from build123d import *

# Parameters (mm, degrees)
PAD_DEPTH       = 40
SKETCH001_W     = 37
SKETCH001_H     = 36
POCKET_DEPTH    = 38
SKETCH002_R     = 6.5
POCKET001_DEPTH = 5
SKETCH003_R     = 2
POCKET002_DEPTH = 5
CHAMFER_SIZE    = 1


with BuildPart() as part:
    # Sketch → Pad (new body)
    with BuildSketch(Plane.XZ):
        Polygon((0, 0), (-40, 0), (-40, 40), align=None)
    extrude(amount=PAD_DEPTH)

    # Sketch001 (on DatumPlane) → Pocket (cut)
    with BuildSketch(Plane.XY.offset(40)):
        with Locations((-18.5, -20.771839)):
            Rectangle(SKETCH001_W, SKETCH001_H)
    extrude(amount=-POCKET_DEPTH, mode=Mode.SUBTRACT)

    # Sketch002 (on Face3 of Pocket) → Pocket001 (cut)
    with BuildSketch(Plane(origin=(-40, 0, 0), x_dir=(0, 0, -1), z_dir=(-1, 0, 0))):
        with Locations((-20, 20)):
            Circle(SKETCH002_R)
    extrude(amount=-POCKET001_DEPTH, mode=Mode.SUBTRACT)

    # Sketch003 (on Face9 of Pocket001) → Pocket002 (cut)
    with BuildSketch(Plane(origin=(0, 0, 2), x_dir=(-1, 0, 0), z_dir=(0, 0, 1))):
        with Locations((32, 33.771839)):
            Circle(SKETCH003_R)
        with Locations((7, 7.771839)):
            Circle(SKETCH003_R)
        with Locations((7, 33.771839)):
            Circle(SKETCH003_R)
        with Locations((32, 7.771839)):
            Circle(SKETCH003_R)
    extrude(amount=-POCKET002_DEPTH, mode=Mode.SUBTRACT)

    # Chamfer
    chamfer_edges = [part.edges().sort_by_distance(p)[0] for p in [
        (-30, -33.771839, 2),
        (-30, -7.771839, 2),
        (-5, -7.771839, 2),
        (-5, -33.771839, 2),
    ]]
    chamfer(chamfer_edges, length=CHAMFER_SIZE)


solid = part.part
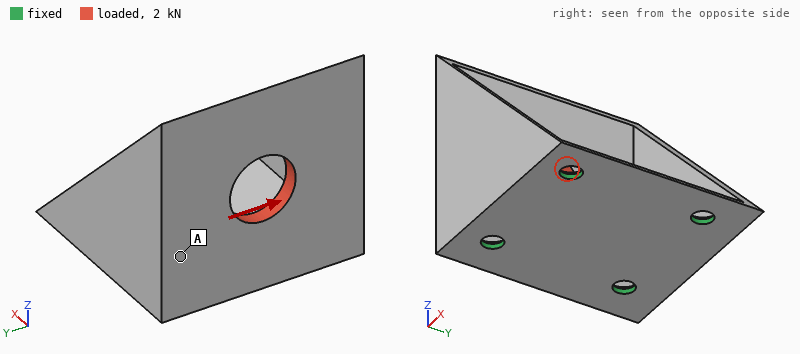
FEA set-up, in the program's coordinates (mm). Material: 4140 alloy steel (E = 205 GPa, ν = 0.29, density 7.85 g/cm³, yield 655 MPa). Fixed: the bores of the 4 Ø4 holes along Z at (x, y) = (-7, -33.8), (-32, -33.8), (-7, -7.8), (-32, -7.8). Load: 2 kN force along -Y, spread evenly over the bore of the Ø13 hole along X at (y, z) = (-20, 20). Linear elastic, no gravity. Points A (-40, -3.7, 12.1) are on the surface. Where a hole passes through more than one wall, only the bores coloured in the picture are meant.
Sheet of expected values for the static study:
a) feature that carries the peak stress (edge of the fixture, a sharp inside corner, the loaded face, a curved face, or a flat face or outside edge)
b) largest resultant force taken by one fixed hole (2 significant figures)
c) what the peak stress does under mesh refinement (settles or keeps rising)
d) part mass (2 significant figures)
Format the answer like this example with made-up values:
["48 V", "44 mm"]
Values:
["edge of the fixture", "1.9 kN", "keeps rising", "74 g"]
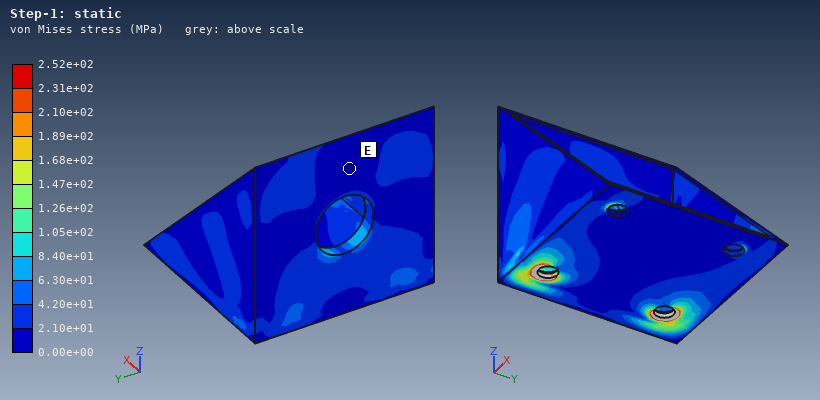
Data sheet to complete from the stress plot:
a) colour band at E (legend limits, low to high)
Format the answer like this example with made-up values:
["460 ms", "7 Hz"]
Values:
["0.00e+00 to 2.10e+01 MPa"]
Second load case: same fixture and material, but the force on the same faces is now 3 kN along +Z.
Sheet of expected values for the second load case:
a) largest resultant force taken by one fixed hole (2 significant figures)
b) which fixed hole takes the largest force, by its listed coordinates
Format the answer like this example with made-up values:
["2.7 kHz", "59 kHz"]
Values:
["1.9 kN", "(-32, -7.8)"]
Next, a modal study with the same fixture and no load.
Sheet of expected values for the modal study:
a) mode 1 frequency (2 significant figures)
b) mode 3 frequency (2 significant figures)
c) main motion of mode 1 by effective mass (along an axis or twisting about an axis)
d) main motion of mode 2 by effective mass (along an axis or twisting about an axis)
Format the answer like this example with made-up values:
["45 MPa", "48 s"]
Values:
["4000 Hz", "6200 Hz", "along X", "along Y"]
